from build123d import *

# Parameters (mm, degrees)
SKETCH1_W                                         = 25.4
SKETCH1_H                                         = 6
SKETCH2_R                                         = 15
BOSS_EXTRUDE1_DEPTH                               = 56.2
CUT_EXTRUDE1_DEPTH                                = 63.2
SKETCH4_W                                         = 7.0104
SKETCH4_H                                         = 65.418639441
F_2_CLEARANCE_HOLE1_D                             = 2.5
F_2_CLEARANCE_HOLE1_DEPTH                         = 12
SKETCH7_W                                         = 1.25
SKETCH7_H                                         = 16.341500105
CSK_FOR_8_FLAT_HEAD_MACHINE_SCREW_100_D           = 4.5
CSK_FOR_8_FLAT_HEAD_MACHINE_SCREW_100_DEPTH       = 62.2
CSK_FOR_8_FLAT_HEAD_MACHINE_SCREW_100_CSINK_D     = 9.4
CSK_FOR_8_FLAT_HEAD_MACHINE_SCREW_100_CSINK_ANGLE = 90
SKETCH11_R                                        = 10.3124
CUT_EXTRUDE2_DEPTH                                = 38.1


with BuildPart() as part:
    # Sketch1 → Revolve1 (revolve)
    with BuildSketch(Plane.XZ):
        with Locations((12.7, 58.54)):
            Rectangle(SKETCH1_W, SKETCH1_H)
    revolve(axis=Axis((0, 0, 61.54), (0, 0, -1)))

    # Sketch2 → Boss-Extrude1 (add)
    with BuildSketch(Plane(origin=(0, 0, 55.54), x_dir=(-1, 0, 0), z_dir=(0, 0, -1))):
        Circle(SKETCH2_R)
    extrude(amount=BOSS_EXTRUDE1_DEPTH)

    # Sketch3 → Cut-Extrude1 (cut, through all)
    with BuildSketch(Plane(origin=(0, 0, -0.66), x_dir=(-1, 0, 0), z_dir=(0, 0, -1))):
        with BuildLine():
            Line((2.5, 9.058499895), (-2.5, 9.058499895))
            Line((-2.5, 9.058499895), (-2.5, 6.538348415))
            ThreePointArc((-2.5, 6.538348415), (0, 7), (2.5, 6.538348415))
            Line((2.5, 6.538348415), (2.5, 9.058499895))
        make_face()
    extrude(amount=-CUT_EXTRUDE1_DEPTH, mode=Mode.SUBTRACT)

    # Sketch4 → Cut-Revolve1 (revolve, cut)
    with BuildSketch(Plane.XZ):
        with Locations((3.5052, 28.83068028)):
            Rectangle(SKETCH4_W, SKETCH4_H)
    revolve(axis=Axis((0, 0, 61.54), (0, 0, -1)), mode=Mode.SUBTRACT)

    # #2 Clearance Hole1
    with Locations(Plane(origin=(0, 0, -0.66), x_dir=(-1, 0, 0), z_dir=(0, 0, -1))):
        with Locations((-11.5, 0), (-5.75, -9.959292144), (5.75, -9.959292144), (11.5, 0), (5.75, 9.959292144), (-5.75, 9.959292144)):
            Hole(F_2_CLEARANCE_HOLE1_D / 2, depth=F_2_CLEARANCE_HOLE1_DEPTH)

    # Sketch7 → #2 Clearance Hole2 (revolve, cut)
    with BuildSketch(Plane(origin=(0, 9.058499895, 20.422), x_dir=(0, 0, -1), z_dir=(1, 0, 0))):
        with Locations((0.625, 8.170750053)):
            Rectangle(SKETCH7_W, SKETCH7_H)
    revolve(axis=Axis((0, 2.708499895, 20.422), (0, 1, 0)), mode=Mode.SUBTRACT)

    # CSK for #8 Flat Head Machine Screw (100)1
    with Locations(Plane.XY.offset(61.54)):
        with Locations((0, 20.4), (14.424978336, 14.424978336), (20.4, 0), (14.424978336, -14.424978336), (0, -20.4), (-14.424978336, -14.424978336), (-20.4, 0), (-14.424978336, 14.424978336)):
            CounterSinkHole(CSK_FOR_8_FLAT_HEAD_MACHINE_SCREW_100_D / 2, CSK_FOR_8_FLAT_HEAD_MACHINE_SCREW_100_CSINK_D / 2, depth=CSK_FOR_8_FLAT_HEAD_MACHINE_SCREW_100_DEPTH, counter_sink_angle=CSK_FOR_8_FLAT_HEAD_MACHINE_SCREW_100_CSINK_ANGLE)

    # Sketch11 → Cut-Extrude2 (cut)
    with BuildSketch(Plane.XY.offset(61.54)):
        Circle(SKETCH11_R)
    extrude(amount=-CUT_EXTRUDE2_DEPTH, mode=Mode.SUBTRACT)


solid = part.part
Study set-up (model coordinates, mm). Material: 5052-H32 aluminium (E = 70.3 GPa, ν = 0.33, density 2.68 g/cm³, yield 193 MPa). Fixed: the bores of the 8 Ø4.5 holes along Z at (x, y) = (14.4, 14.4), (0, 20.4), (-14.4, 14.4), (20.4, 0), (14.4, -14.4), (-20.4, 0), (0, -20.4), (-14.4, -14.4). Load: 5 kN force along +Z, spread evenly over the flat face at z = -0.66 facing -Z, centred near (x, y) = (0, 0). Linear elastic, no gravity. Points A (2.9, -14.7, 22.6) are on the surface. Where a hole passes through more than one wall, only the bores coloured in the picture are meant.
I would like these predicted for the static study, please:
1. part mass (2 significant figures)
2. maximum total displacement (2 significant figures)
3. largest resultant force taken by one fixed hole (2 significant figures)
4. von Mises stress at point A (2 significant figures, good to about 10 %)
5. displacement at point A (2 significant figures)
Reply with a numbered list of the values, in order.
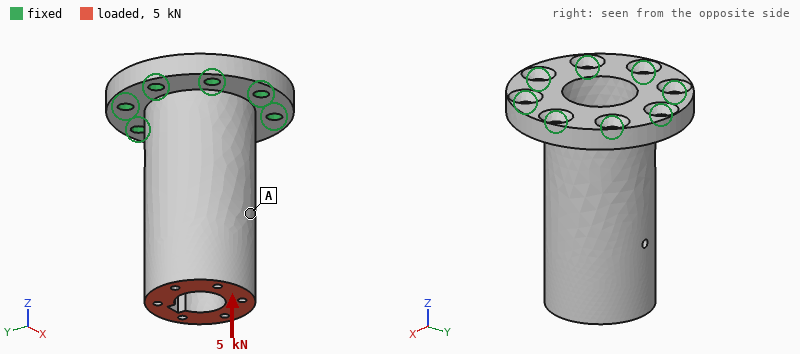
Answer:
1. 90 g
2. 15 µm
3. 650 N
4. 12 MPa
5. 12 µm
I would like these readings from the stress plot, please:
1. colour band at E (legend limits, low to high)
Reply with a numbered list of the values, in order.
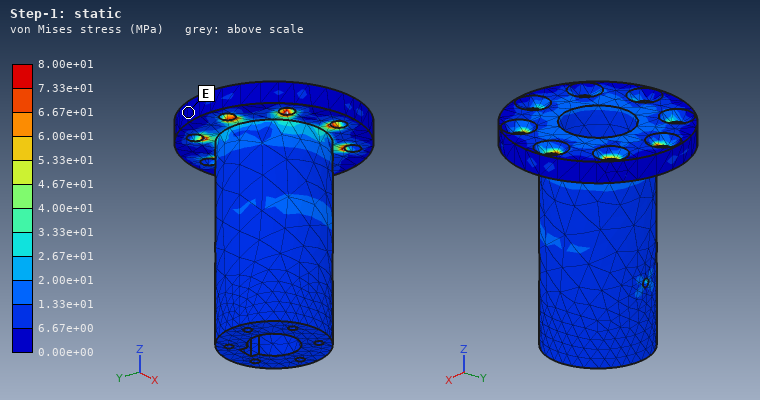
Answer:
1. 0.00e+00 to 6.67e+00 MPa
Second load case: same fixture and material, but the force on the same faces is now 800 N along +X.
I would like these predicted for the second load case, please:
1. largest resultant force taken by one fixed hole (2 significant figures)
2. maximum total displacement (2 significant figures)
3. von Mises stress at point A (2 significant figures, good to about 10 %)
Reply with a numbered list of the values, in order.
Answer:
1. 690 N
2. 50 µm
3. 5.5 MPa
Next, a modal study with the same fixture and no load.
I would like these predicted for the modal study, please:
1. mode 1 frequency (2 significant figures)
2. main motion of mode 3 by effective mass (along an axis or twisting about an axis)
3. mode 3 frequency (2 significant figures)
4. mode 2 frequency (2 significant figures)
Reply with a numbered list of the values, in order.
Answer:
1. 4200 Hz
2. twisting about Z
3. 12 kHz
4. 4200 Hz
